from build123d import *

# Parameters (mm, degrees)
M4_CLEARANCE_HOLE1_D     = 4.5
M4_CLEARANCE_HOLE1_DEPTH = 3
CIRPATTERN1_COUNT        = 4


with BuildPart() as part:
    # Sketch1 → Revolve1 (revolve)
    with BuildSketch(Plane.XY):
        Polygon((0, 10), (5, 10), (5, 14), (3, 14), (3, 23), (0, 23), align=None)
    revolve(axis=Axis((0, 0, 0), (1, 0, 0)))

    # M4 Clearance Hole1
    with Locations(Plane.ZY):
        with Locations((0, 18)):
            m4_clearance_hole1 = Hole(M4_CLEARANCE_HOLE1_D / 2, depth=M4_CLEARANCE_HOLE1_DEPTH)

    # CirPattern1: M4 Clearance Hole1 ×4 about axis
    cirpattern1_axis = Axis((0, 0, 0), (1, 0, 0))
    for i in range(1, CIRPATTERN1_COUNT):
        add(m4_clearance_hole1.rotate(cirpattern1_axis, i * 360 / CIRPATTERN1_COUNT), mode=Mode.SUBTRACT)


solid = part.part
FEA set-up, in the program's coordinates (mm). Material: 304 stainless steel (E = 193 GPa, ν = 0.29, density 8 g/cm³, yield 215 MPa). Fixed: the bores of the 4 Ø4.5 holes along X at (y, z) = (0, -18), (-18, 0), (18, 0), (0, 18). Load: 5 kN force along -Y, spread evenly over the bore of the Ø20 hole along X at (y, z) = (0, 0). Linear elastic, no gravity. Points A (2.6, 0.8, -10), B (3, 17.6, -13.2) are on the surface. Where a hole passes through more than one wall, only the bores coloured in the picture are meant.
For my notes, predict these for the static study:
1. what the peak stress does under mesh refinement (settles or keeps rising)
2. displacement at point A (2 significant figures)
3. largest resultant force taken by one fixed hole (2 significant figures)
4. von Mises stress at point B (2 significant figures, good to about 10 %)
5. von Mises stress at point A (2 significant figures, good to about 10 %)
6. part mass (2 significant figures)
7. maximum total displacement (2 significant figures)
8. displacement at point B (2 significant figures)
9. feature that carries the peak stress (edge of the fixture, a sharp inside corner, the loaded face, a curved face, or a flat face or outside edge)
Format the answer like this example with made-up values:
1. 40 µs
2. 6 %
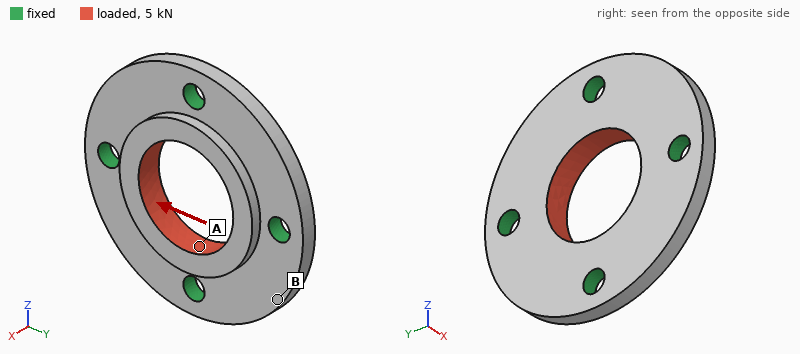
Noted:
1. keeps rising
2. 2.3 µm
3. 1.3 kN
4. 12 MPa
5. 34 MPa
6. 36 g
7. 3.0 µm
8. 1.9 µm
9. edge of the fixture
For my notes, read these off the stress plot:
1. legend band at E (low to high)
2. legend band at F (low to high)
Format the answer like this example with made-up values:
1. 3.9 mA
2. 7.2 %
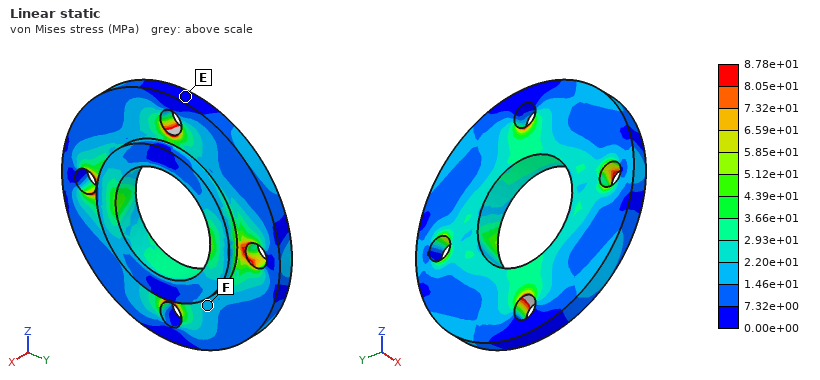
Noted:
1. 0.00e+00 to 7.32e+00 MPa
2. 1.46e+01 to 2.20e+01 MPa
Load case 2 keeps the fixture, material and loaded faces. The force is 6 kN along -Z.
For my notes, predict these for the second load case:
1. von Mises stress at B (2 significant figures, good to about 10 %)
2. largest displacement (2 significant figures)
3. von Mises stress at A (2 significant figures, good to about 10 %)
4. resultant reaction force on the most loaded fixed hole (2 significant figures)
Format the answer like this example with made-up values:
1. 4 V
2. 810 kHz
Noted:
1. 16 MPa
2. 3.7 µm
3. 52 MPa
4. 1.6 kN
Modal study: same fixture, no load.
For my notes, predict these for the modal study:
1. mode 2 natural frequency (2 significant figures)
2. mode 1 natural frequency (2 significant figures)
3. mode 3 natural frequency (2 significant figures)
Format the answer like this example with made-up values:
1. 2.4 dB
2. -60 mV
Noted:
1. 21 kHz
2. 20 kHz
3. 21 kHz
